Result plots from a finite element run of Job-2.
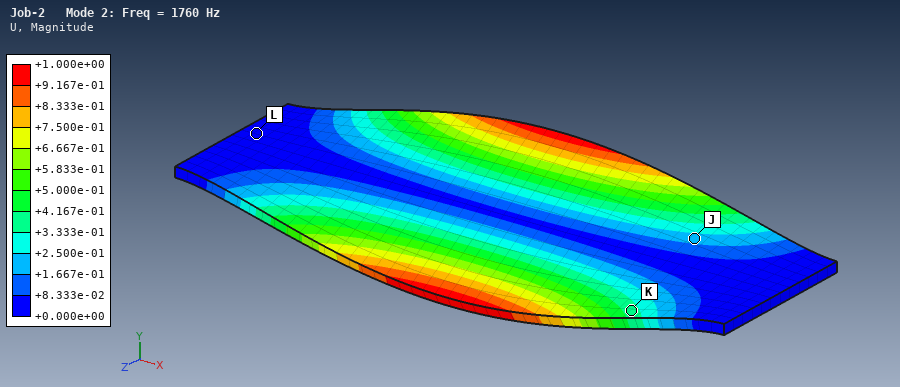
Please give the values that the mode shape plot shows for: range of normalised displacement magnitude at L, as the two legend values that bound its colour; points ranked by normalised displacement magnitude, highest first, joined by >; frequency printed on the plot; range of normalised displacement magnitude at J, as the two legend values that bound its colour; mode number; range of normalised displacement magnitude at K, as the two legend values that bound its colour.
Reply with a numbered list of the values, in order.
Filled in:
1. +0.000e+00 to +8.333e-02
2. K > J > L
3. 1760 Hz
4. +1.667e-01 to +2.500e-01
5. 2
6. +3.333e-01 to +4.167e-01
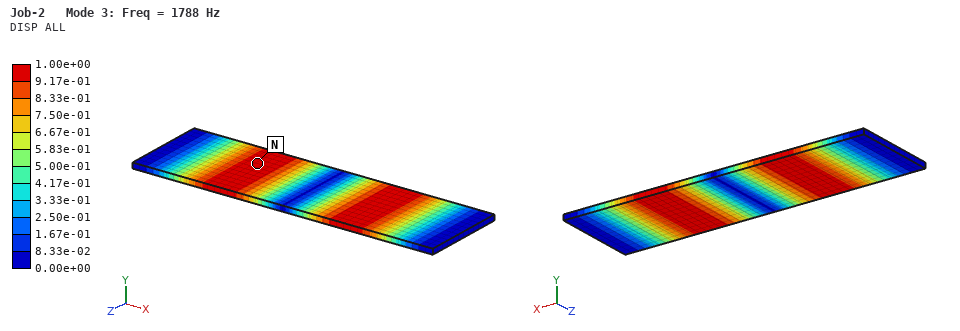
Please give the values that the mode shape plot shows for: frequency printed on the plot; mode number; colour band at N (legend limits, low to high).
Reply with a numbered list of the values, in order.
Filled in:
1. 1788 Hz
2. 3
3. 9.17e-01 to 1.00e+00
